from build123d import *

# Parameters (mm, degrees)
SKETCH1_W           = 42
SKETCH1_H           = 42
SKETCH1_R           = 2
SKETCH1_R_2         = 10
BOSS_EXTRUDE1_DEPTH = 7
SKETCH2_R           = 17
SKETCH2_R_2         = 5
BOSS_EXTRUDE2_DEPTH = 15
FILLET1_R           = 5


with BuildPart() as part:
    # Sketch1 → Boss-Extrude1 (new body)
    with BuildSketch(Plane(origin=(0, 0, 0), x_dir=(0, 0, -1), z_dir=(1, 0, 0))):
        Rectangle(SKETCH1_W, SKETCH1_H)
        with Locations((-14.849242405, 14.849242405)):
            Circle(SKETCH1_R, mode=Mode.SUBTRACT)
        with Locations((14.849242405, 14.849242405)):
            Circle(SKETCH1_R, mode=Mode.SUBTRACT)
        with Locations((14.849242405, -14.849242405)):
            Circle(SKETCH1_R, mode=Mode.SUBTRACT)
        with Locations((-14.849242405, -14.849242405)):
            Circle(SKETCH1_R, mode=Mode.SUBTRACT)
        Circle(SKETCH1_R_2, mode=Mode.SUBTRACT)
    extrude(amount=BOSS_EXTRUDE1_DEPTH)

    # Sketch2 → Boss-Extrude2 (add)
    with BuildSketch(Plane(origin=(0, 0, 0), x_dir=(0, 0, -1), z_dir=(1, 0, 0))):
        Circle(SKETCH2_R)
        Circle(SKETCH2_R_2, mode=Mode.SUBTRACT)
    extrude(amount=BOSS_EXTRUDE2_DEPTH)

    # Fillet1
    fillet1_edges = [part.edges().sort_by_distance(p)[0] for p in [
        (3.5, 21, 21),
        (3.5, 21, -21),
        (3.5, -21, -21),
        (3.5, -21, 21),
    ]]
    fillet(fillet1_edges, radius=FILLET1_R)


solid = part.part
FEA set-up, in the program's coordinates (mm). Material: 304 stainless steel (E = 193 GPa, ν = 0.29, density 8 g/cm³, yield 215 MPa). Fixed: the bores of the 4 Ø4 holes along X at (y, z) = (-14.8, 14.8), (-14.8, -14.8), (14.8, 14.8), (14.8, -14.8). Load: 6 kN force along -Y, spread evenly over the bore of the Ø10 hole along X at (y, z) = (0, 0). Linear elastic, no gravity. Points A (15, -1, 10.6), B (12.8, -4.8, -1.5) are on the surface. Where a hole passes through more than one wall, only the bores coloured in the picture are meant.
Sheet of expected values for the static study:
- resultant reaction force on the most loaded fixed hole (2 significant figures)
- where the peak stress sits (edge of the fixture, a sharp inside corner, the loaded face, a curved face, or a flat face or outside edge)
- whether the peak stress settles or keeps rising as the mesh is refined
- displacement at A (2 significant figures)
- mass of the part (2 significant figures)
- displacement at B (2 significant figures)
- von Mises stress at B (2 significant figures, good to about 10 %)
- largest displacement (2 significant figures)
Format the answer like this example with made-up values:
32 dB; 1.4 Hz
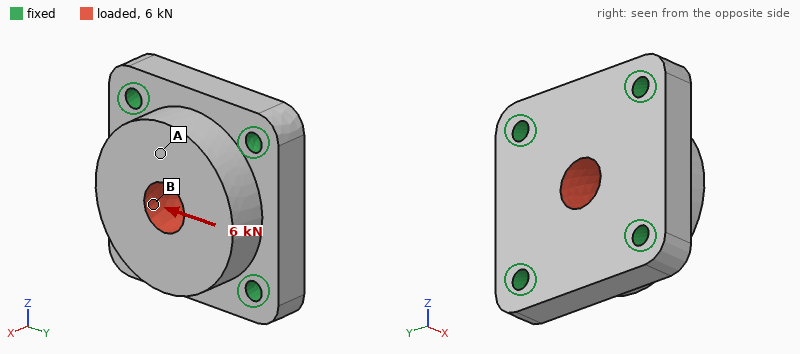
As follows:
1.7 kN; edge of the fixture; keeps rising; 1.5 µm; 140 g; 2.2 µm; 13 MPa; 2.3 µm
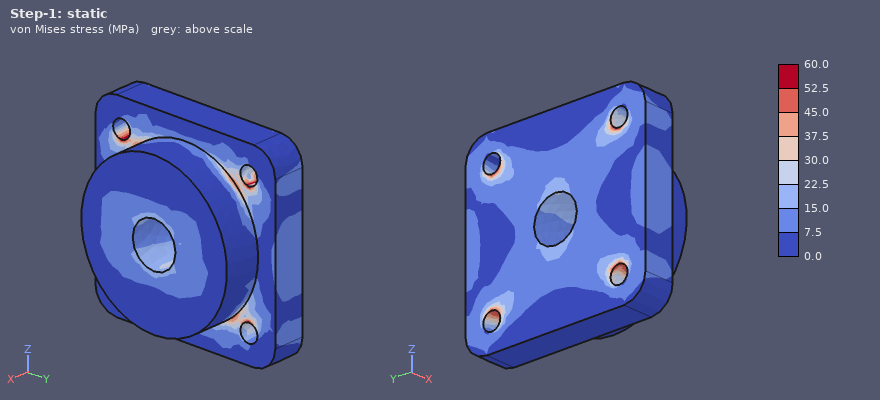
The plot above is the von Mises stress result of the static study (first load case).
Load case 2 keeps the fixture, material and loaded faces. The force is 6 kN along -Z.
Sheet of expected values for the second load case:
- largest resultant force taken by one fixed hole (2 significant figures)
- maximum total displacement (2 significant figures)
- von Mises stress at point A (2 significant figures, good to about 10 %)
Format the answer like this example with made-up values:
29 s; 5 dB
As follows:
1.7 kN; 2.3 µm; 8.3 MPa
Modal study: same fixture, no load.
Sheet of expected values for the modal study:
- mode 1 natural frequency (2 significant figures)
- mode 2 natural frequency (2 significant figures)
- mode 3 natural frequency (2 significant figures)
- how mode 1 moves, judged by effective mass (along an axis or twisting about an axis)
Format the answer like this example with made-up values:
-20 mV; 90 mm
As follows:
24 kHz; 29 kHz; 29 kHz; along X
